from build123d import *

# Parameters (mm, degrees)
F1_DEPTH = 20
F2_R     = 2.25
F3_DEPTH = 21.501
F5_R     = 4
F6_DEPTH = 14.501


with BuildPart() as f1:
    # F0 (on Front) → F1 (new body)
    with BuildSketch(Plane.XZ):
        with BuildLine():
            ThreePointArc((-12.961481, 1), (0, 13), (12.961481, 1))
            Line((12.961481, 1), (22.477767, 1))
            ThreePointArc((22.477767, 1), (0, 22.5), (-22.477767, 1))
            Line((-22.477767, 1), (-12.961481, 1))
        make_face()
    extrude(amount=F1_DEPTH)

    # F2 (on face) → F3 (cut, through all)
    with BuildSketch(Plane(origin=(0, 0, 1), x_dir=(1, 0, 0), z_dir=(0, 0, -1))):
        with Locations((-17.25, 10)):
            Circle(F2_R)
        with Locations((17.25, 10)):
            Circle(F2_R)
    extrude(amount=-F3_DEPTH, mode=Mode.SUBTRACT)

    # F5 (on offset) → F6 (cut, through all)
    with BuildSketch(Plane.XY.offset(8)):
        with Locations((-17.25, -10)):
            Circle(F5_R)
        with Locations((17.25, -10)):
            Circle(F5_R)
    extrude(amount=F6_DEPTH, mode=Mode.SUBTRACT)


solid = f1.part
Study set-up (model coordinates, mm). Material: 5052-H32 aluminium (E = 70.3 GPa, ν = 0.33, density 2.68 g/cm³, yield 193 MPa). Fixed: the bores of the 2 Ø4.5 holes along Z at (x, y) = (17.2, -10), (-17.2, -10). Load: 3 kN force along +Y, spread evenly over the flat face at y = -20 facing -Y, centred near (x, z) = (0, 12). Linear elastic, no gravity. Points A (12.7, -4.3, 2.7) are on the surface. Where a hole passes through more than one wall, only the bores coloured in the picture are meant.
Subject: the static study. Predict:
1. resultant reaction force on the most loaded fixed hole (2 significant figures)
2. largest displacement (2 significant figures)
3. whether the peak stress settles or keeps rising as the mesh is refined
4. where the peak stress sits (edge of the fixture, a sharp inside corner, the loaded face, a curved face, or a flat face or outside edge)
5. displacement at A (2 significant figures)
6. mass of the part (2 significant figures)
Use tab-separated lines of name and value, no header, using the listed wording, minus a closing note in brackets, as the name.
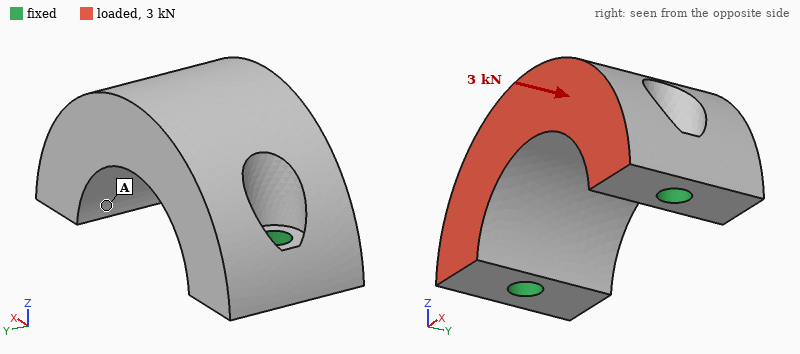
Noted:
resultant reaction force on the most loaded fixed hole	1.5 kN
largest displacement	31 µm
whether the peak stress settles or keeps rising as the mesh is refined	keeps rising
where the peak stress sits	edge of the fixture
displacement at A	5.0 µm
mass of the part	25 g
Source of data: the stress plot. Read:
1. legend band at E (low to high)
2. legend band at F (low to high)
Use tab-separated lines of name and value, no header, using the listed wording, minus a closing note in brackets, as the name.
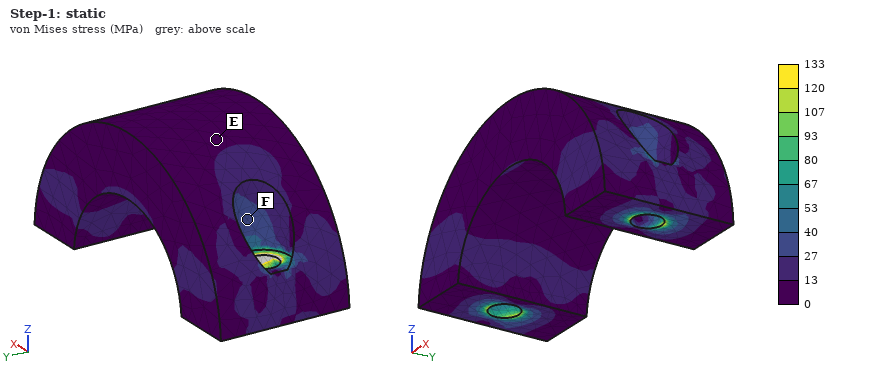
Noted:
legend band at E	0 to 13 MPa
legend band at F	27 to 40 MPa
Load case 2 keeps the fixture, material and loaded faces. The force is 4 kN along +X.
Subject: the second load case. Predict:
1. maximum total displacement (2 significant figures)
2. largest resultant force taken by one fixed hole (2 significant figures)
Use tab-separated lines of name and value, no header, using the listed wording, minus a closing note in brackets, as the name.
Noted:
maximum total displacement	20 µm
largest resultant force taken by one fixed hole	2.3 kN
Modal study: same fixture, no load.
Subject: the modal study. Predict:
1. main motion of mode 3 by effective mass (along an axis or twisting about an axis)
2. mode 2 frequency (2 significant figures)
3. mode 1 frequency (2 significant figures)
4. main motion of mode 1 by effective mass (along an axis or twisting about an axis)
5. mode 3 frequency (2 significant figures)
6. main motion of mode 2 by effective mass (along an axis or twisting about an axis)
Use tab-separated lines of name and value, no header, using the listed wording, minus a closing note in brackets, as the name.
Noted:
main motion of mode 3 by effective mass	twisting about Z
mode 2 frequency	24 kHz
mode 1 frequency	12 kHz
main motion of mode 1 by effective mass	along Y
mode 3 frequency	28 kHz
main motion of mode 2 by effective mass	along X
